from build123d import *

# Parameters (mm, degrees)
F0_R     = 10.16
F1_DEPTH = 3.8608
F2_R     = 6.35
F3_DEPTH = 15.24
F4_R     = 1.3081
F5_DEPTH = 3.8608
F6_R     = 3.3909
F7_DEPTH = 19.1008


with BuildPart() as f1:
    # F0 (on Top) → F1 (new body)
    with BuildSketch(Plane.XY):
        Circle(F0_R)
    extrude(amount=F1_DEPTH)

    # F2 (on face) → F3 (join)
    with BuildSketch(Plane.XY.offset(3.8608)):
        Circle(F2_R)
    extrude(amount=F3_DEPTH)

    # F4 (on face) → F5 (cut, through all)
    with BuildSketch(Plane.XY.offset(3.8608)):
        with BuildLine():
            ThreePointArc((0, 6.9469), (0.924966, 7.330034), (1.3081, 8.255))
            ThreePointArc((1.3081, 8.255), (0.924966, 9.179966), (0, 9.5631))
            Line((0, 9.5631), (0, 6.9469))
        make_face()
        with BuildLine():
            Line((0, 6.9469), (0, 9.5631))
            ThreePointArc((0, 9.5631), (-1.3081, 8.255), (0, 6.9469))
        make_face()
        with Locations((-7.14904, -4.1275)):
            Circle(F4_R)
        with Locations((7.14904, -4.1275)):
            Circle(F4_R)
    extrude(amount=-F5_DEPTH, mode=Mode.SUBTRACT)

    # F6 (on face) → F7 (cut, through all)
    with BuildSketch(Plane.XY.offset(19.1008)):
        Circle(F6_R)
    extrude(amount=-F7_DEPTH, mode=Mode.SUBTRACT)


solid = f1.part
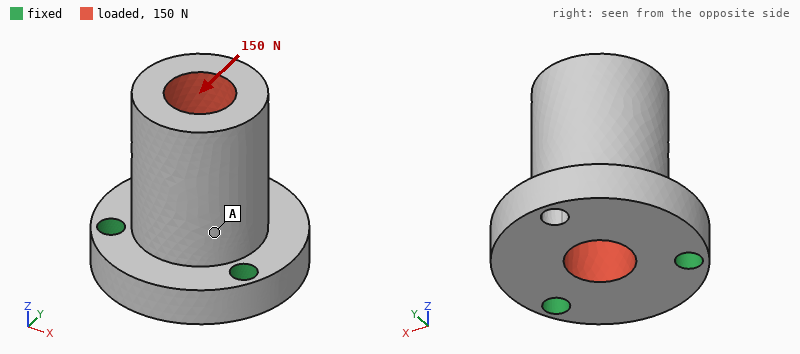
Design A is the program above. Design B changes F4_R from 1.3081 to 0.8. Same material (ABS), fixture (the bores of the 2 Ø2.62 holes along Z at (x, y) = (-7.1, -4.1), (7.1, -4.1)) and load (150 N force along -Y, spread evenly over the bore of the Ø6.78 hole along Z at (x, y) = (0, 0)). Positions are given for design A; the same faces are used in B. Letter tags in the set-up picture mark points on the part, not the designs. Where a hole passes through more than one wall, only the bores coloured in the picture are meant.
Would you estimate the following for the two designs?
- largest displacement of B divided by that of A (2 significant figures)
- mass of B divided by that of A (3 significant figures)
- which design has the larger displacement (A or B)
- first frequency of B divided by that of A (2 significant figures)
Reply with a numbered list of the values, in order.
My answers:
1. 1.3
2. 1.01
3. B
4. 0.85
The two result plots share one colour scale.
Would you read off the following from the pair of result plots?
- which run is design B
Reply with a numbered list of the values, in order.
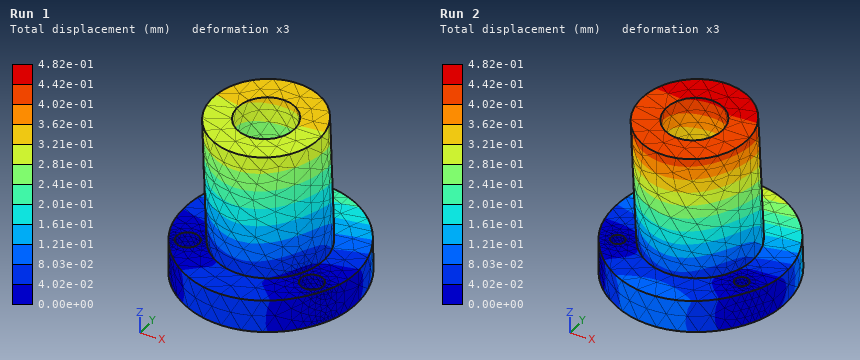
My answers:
1. Run 2
